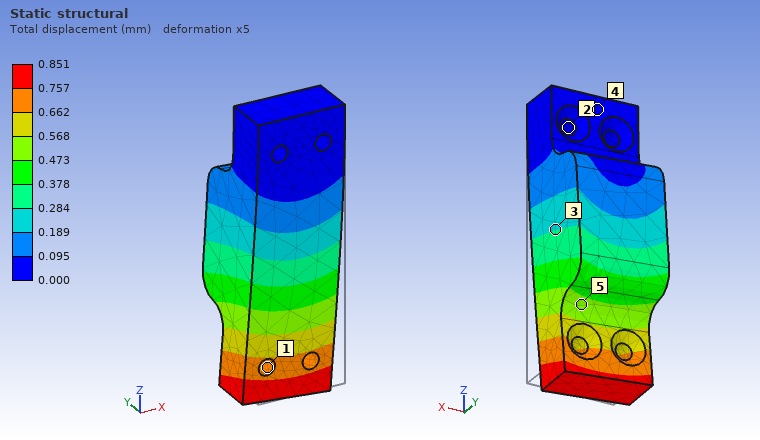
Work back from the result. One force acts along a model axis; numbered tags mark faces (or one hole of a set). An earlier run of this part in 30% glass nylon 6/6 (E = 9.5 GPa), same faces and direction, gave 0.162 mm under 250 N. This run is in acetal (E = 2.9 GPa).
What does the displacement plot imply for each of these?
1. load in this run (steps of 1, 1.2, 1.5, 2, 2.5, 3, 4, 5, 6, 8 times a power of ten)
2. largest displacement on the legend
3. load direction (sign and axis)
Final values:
400 N
0.851 mm
-X
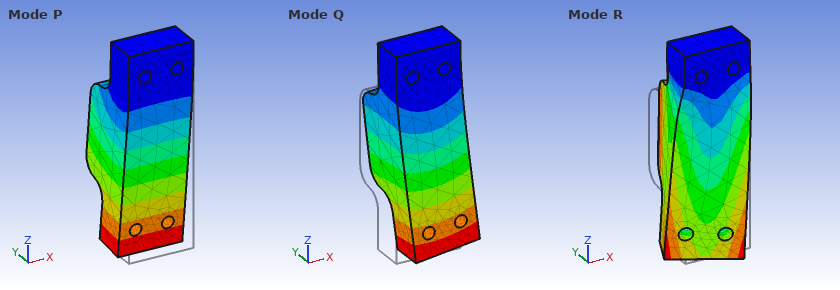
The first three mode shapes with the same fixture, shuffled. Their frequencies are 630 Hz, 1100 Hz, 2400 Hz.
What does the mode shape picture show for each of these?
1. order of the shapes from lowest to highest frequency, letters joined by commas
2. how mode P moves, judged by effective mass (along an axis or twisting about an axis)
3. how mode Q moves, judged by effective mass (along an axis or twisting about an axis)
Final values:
P, Q, R
along Y
along X
